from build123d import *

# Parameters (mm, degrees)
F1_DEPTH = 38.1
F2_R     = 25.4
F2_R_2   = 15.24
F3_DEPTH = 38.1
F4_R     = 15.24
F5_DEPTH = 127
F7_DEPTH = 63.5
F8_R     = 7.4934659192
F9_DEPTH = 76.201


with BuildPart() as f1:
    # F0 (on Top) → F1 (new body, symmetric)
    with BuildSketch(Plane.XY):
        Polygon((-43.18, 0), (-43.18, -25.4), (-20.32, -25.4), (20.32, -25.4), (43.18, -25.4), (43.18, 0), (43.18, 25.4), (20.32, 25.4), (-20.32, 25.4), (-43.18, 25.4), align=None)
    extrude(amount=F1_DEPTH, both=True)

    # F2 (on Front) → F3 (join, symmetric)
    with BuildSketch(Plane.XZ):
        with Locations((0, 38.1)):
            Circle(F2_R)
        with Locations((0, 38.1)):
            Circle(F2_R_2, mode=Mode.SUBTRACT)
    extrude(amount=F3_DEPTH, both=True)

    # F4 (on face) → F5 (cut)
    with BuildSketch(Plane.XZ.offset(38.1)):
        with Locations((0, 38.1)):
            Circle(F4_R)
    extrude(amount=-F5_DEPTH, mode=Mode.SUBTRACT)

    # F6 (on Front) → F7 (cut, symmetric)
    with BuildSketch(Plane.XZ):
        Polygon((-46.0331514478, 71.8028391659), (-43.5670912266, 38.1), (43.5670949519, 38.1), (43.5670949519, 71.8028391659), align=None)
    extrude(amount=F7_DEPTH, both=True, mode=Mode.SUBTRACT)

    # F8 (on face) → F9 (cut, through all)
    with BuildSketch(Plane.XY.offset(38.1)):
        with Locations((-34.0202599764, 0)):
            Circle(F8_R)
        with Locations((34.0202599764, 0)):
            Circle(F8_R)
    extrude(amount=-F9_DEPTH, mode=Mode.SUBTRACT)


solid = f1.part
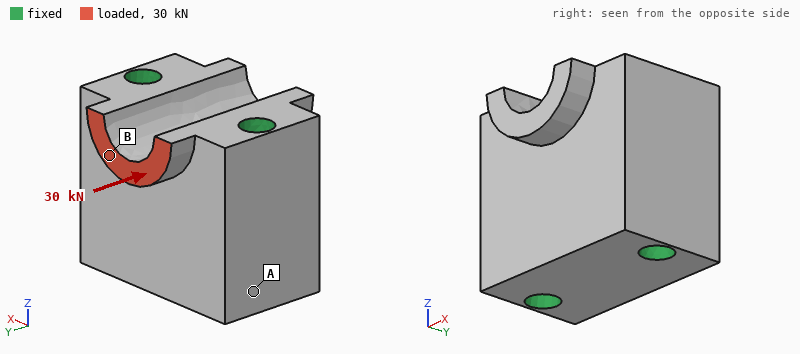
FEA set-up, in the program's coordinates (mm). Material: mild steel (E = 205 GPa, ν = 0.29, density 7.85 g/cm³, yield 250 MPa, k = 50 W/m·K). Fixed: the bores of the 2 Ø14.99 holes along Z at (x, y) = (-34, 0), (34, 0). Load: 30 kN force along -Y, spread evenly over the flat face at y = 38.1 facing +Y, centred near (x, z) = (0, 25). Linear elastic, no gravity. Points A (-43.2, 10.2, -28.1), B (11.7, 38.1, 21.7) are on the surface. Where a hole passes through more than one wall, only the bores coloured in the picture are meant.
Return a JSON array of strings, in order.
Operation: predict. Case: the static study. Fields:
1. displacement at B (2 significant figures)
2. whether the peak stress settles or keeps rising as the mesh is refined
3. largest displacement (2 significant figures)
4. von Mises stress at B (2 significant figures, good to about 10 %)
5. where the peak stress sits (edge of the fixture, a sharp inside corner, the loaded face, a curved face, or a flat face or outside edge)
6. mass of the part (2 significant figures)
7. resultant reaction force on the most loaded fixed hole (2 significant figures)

["7.2 µm", "keeps rising", "10 µm", "43 MPa", "a sharp inside corner", "2.4 kg", "16 kN"]
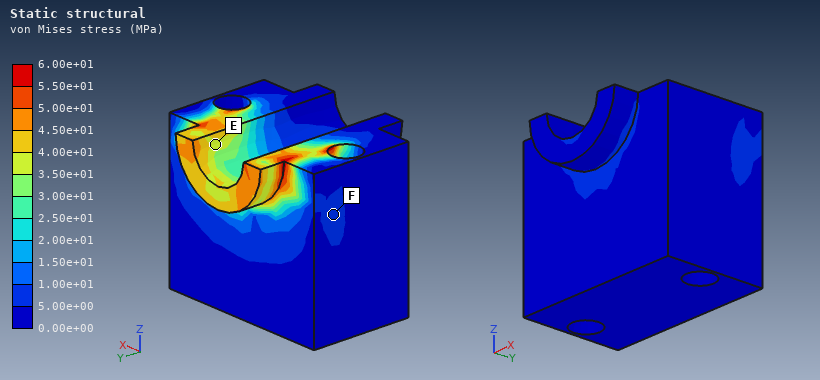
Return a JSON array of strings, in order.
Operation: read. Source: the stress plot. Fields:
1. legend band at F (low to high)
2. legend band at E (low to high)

["5.00e+00 to 1.00e+01 MPa", "3.50e+01 to 4.00e+01 MPa"]
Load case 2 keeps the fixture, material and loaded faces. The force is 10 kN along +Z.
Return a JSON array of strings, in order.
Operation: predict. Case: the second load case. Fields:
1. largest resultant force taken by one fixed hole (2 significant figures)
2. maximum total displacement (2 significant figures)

["5.0 kN", "16 µm"]
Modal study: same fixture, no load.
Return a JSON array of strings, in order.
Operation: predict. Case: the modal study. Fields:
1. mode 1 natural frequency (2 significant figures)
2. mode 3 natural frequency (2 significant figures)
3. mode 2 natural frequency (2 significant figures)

["20 kHz", "20 kHz", "20 kHz"]
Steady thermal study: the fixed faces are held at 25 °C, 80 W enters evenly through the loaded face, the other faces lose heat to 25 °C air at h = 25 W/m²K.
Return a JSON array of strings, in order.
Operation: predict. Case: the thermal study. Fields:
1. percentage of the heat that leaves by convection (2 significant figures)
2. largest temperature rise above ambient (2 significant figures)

["4.5 %", "56 K"]
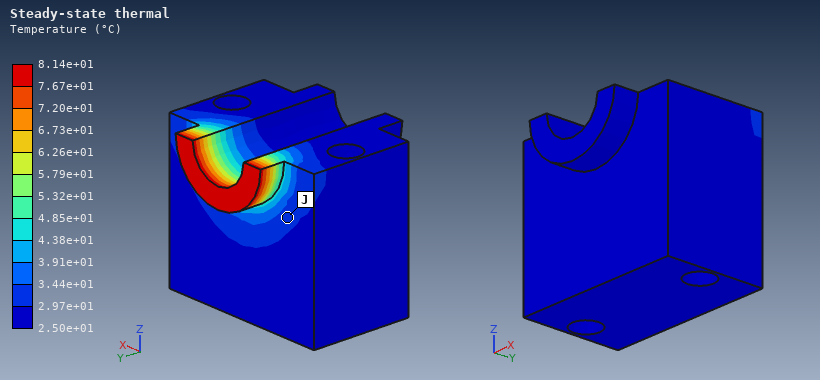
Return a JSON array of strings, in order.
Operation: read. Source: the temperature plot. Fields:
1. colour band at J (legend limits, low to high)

["2.97e+01 to 3.44e+01 °C"]
